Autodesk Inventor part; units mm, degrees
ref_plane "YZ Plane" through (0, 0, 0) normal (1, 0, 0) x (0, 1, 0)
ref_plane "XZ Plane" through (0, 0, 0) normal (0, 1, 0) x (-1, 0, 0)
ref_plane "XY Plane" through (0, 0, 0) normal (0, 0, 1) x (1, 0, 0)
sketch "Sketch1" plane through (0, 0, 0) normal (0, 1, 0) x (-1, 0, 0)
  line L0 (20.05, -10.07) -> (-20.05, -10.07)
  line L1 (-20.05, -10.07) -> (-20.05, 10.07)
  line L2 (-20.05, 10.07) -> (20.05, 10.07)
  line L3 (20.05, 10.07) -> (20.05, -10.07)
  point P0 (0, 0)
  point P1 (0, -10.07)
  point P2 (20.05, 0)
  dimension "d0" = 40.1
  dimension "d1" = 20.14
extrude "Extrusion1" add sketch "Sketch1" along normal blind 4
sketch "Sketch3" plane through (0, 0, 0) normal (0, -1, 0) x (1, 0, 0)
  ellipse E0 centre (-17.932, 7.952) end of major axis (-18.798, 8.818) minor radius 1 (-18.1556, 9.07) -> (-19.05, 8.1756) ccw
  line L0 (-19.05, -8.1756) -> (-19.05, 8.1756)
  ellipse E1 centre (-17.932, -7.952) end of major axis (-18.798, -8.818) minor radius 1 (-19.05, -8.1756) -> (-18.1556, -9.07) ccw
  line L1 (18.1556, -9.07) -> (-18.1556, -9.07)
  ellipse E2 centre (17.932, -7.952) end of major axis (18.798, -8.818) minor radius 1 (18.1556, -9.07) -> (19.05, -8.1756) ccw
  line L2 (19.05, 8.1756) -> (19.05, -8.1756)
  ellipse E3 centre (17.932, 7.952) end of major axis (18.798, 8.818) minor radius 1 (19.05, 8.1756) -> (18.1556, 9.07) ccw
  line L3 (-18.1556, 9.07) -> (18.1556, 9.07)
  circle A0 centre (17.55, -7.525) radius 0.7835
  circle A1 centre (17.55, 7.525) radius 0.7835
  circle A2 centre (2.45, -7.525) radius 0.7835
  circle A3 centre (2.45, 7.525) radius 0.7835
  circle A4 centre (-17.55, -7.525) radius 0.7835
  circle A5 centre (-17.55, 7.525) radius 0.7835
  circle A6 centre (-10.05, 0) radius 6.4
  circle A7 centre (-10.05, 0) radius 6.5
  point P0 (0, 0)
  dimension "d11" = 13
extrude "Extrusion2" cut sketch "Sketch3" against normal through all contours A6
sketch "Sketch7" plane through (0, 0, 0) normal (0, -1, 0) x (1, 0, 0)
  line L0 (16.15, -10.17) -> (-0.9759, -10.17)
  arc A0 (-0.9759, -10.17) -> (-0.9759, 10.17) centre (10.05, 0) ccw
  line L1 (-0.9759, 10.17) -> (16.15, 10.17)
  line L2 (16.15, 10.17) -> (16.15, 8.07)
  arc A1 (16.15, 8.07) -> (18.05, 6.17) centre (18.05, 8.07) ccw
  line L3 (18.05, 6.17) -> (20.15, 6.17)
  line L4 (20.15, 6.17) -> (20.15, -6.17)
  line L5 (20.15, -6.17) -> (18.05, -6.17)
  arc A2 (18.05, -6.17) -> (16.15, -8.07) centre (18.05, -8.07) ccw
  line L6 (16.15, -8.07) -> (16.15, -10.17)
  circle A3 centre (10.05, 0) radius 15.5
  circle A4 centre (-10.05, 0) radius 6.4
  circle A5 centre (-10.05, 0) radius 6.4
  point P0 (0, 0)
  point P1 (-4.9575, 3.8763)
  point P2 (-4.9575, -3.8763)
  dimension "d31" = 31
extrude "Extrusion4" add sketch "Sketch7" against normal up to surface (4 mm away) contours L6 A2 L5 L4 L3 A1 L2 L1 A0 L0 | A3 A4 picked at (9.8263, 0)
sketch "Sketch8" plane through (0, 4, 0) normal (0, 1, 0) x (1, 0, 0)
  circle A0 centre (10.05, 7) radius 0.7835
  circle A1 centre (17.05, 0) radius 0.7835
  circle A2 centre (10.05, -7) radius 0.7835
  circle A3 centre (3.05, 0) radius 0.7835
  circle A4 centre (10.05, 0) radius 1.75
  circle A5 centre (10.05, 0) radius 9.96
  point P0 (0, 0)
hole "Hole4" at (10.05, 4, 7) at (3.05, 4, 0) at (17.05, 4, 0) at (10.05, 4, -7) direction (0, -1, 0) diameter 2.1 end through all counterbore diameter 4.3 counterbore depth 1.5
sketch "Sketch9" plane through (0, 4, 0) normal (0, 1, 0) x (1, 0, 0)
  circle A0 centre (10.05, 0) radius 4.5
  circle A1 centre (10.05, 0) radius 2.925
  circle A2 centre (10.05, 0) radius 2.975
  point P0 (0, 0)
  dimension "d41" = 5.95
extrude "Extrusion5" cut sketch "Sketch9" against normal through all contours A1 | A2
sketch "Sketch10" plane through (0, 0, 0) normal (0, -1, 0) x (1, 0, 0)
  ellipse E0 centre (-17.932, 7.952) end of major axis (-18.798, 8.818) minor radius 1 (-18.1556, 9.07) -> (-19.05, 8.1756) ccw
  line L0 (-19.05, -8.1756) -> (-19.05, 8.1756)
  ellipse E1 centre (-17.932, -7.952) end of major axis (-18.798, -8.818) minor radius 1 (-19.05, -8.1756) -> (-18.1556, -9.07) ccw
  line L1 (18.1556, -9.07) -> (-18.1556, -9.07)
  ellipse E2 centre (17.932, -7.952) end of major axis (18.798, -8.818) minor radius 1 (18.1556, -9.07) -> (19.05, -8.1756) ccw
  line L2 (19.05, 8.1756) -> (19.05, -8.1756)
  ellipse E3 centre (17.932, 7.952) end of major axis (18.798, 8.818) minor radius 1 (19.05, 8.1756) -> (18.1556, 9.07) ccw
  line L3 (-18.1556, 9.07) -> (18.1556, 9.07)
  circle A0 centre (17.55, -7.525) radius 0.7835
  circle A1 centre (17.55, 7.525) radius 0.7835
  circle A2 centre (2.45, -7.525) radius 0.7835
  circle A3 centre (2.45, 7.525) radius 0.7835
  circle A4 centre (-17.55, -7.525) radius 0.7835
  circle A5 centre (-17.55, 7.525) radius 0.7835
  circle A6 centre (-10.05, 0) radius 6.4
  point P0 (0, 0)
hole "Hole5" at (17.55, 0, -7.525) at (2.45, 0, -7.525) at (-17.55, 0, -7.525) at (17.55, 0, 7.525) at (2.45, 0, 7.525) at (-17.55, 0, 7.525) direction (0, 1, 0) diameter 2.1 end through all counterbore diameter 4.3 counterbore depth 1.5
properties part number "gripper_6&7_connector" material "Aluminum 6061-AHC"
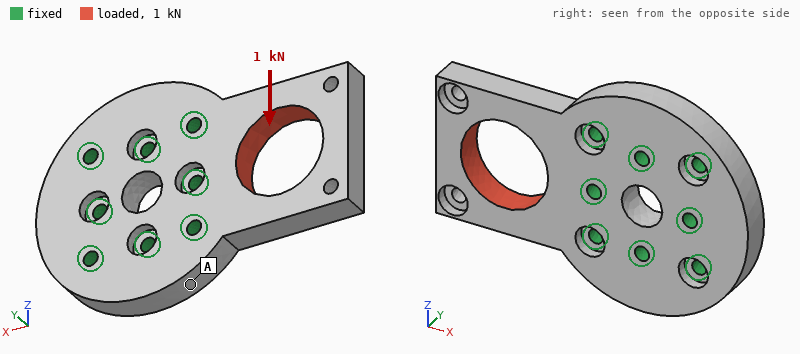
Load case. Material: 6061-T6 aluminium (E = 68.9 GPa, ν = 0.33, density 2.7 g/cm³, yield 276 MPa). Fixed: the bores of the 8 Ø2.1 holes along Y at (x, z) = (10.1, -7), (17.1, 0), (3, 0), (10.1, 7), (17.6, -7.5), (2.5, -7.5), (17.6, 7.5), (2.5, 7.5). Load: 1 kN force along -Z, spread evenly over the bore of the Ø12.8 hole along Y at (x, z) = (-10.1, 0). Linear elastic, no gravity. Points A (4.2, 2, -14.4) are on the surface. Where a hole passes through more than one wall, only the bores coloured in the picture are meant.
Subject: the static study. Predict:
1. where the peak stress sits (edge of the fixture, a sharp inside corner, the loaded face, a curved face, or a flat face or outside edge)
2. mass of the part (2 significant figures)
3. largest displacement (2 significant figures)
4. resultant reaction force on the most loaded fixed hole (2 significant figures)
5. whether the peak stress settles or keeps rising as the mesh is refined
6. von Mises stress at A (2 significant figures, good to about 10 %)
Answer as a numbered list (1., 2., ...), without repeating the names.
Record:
1. edge of the fixture
2. 9.1 g
3. 52 µm
4. 600 N
5. keeps rising
6. 11 MPa
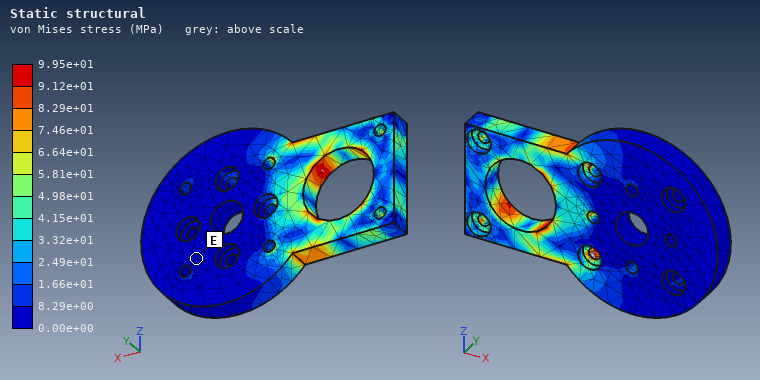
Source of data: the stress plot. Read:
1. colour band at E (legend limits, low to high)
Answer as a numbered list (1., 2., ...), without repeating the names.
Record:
1. 0.00e+00 to 8.29e+00 MPa
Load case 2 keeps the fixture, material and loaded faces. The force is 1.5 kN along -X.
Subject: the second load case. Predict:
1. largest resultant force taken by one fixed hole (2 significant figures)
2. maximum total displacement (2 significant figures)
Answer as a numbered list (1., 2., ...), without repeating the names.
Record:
1. 480 N
2. 18 µm
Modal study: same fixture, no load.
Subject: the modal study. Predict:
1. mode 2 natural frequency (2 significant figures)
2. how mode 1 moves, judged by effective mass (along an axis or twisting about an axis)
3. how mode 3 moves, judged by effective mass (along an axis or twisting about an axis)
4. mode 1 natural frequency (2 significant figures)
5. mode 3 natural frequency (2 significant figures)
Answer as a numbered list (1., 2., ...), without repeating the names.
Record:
1. 13 kHz
2. along Y
3. along Z
4. 5900 Hz
5. 16 kHz
